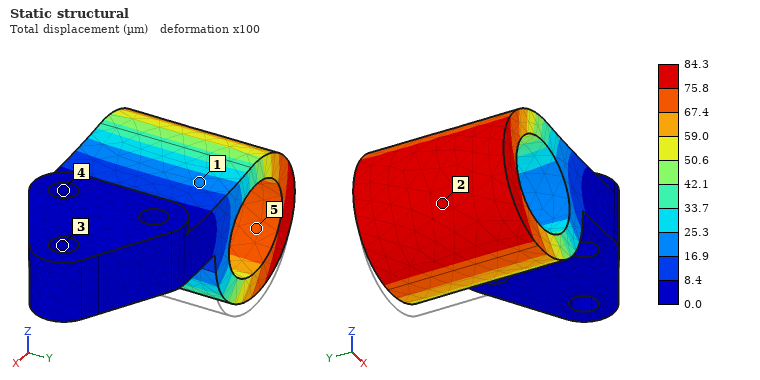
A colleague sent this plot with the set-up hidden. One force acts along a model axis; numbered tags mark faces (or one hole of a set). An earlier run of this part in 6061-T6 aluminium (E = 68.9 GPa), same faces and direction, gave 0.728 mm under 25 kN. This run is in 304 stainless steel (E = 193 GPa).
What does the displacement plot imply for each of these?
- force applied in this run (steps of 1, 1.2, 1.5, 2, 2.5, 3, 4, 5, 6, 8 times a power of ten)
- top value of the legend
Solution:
8 kN
84.3 µm
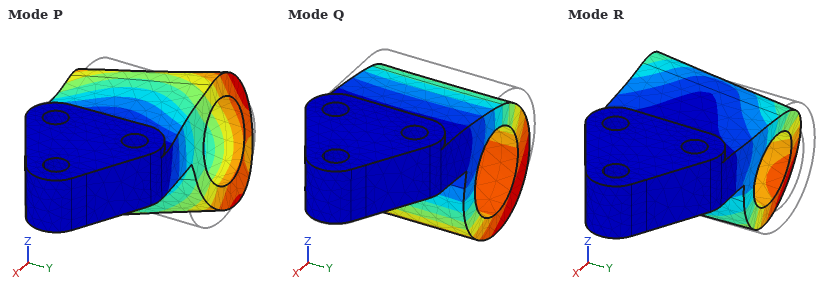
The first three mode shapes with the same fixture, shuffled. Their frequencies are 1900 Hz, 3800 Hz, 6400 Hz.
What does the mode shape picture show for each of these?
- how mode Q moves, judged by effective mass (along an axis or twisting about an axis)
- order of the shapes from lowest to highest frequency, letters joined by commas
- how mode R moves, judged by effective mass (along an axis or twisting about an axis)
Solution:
along Z
Q, R, P
along Y
